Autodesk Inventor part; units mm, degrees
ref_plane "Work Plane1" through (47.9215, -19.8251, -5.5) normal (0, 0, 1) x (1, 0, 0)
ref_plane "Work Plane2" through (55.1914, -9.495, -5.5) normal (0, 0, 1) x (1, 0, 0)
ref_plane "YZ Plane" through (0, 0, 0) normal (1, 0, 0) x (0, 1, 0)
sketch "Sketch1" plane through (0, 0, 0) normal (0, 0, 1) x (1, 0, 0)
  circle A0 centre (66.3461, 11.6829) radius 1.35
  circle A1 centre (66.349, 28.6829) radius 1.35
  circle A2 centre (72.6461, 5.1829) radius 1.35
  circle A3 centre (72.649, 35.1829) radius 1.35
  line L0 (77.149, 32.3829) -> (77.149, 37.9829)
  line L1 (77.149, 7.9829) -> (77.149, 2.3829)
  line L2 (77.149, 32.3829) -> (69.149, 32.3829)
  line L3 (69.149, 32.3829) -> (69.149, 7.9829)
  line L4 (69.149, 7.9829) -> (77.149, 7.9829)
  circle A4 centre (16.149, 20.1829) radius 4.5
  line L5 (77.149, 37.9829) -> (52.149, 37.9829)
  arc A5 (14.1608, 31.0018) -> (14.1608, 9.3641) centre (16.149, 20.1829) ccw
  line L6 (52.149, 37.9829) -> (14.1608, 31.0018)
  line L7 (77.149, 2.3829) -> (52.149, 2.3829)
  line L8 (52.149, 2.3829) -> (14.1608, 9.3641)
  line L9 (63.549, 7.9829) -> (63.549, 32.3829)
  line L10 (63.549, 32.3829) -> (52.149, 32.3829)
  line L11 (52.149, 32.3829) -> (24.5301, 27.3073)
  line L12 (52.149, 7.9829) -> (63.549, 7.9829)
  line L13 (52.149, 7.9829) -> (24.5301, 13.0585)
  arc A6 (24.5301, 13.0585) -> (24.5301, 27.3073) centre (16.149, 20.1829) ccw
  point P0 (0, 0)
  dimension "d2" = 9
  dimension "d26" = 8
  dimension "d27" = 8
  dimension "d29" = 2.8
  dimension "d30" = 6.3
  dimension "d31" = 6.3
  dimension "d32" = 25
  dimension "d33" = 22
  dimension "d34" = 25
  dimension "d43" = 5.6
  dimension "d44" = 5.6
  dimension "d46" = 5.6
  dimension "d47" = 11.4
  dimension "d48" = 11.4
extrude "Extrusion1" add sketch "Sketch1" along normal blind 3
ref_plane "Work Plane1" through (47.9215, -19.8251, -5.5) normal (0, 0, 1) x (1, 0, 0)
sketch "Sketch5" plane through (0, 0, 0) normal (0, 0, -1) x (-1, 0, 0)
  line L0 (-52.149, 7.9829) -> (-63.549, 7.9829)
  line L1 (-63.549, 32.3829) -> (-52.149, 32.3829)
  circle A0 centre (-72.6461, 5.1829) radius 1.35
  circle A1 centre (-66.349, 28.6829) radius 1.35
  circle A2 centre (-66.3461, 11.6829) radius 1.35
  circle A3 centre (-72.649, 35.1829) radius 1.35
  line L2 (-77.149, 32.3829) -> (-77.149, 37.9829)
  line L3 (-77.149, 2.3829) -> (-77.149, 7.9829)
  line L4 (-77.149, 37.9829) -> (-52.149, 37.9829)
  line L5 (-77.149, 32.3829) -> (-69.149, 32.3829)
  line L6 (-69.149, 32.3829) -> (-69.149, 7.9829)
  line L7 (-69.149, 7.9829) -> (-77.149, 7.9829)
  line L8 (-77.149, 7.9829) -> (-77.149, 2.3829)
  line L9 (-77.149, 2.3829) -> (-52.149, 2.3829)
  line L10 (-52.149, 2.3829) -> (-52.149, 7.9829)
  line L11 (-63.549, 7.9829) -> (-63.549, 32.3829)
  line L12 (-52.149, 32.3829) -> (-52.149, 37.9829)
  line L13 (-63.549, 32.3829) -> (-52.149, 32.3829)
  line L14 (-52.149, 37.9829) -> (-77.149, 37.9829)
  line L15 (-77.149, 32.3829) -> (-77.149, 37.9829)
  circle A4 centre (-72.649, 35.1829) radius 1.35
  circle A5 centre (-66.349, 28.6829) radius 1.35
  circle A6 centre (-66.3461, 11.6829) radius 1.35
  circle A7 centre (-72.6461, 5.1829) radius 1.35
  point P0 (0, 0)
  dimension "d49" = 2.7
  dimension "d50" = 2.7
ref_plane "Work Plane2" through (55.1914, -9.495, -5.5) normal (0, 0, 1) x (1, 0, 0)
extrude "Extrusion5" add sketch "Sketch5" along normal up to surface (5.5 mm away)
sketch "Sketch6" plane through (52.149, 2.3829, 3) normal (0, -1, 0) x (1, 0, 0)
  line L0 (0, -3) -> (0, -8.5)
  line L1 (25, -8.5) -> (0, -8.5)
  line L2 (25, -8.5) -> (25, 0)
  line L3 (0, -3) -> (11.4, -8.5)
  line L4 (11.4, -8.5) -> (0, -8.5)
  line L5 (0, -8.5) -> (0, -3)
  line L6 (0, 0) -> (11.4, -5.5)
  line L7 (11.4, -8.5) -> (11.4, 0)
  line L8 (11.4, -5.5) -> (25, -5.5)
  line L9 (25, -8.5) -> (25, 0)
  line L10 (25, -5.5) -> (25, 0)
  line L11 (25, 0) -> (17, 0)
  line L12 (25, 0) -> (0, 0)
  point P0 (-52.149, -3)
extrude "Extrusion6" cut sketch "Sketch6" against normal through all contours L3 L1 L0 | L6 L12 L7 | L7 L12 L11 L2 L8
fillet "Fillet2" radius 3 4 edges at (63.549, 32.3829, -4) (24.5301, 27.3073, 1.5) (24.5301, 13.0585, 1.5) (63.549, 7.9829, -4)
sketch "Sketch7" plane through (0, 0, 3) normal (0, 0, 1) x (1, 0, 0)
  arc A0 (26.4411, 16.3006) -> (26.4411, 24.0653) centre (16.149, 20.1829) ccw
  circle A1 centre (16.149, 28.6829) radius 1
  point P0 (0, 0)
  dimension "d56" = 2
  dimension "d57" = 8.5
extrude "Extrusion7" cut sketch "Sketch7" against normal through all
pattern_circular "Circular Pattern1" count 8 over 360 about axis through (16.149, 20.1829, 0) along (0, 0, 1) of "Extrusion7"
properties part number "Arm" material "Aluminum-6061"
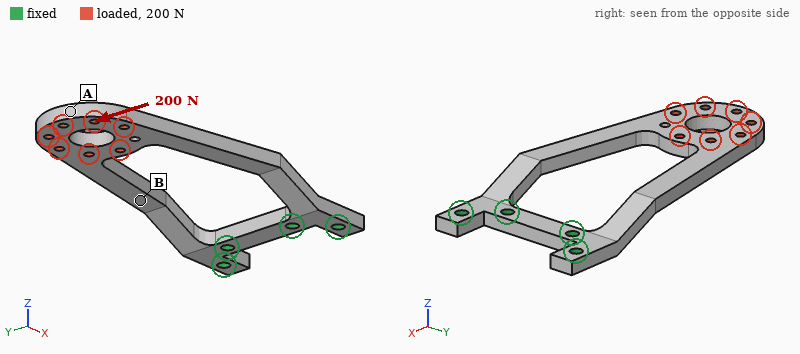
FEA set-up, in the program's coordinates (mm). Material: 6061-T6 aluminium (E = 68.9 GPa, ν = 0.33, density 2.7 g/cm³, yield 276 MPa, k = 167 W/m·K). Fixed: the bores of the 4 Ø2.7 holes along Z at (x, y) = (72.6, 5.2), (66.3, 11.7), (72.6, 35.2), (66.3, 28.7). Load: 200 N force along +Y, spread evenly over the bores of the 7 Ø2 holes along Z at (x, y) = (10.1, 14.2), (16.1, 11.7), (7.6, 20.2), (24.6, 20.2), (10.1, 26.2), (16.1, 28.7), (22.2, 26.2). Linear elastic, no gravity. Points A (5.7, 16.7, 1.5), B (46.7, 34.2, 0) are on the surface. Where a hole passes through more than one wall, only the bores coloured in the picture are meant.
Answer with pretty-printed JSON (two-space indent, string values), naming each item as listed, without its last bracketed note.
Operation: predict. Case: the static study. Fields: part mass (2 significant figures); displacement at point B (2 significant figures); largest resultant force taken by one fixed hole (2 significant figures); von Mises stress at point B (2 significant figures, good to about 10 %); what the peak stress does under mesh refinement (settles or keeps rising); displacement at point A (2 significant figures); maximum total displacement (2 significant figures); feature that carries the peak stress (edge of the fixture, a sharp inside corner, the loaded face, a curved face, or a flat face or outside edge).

{
  "part mass": "8.4 g",
  "displacement at point B": "0.13 mm",
  "largest resultant force taken by one fixed hole": "400 N",
  "von Mises stress at point B": "60 MPa",
  "what the peak stress does under mesh refinement": "keeps rising",
  "displacement at point A": "0.24 mm",
  "maximum total displacement": "0.26 mm",
  "feature that carries the peak stress": "a sharp inside corner"
}
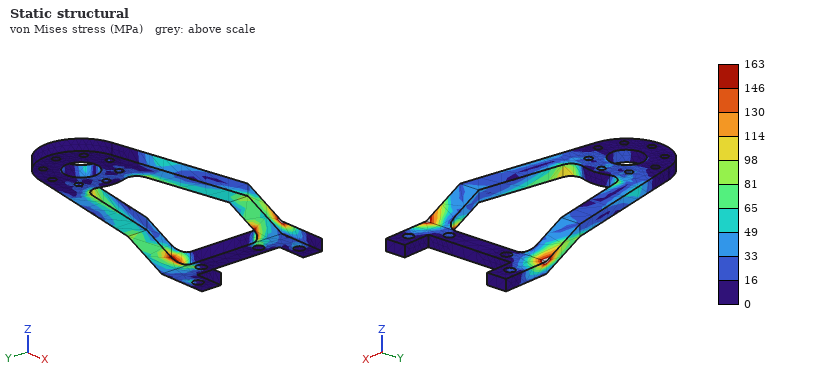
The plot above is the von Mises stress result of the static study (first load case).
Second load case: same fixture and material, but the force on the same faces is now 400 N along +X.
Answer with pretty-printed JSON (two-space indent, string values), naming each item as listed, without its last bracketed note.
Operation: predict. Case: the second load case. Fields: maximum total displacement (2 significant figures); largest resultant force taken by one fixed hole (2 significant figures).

{
  "maximum total displacement": "0.81 mm",
  "largest resultant force taken by one fixed hole": "230 N"
}
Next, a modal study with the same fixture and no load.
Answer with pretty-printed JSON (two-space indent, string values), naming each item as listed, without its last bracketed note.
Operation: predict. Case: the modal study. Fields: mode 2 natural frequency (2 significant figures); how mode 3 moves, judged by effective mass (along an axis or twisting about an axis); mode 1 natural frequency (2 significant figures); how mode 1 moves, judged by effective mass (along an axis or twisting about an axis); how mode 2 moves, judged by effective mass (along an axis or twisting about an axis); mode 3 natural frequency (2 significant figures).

{
  "mode 2 natural frequency": "2100 Hz",
  "how mode 3 moves, judged by effective mass": "along Y",
  "mode 1 natural frequency": "510 Hz",
  "how mode 1 moves, judged by effective mass": "along Z",
  "how mode 2 moves, judged by effective mass": "along Y",
  "mode 3 natural frequency": "2900 Hz"
}
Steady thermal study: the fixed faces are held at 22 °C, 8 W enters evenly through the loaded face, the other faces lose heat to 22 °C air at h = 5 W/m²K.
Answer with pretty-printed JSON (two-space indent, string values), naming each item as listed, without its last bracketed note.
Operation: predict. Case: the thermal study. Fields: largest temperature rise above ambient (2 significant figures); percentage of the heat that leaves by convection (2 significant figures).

{
  "largest temperature rise above ambient": "73 K",
  "percentage of the heat that leaves by convection": "7.0 %"
}
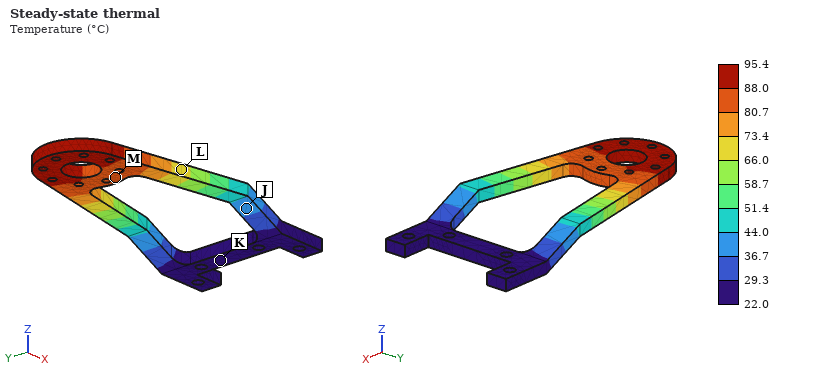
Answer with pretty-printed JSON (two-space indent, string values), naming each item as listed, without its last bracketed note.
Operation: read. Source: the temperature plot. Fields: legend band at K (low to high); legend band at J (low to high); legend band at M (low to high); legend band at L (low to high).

{
  "legend band at K": "22.0 to 29.3 °C",
  "legend band at J": "36.7 to 44.0 °C",
  "legend band at M": "80.7 to 88.0 °C",
  "legend band at L": "66.0 to 73.4 °C"
}
